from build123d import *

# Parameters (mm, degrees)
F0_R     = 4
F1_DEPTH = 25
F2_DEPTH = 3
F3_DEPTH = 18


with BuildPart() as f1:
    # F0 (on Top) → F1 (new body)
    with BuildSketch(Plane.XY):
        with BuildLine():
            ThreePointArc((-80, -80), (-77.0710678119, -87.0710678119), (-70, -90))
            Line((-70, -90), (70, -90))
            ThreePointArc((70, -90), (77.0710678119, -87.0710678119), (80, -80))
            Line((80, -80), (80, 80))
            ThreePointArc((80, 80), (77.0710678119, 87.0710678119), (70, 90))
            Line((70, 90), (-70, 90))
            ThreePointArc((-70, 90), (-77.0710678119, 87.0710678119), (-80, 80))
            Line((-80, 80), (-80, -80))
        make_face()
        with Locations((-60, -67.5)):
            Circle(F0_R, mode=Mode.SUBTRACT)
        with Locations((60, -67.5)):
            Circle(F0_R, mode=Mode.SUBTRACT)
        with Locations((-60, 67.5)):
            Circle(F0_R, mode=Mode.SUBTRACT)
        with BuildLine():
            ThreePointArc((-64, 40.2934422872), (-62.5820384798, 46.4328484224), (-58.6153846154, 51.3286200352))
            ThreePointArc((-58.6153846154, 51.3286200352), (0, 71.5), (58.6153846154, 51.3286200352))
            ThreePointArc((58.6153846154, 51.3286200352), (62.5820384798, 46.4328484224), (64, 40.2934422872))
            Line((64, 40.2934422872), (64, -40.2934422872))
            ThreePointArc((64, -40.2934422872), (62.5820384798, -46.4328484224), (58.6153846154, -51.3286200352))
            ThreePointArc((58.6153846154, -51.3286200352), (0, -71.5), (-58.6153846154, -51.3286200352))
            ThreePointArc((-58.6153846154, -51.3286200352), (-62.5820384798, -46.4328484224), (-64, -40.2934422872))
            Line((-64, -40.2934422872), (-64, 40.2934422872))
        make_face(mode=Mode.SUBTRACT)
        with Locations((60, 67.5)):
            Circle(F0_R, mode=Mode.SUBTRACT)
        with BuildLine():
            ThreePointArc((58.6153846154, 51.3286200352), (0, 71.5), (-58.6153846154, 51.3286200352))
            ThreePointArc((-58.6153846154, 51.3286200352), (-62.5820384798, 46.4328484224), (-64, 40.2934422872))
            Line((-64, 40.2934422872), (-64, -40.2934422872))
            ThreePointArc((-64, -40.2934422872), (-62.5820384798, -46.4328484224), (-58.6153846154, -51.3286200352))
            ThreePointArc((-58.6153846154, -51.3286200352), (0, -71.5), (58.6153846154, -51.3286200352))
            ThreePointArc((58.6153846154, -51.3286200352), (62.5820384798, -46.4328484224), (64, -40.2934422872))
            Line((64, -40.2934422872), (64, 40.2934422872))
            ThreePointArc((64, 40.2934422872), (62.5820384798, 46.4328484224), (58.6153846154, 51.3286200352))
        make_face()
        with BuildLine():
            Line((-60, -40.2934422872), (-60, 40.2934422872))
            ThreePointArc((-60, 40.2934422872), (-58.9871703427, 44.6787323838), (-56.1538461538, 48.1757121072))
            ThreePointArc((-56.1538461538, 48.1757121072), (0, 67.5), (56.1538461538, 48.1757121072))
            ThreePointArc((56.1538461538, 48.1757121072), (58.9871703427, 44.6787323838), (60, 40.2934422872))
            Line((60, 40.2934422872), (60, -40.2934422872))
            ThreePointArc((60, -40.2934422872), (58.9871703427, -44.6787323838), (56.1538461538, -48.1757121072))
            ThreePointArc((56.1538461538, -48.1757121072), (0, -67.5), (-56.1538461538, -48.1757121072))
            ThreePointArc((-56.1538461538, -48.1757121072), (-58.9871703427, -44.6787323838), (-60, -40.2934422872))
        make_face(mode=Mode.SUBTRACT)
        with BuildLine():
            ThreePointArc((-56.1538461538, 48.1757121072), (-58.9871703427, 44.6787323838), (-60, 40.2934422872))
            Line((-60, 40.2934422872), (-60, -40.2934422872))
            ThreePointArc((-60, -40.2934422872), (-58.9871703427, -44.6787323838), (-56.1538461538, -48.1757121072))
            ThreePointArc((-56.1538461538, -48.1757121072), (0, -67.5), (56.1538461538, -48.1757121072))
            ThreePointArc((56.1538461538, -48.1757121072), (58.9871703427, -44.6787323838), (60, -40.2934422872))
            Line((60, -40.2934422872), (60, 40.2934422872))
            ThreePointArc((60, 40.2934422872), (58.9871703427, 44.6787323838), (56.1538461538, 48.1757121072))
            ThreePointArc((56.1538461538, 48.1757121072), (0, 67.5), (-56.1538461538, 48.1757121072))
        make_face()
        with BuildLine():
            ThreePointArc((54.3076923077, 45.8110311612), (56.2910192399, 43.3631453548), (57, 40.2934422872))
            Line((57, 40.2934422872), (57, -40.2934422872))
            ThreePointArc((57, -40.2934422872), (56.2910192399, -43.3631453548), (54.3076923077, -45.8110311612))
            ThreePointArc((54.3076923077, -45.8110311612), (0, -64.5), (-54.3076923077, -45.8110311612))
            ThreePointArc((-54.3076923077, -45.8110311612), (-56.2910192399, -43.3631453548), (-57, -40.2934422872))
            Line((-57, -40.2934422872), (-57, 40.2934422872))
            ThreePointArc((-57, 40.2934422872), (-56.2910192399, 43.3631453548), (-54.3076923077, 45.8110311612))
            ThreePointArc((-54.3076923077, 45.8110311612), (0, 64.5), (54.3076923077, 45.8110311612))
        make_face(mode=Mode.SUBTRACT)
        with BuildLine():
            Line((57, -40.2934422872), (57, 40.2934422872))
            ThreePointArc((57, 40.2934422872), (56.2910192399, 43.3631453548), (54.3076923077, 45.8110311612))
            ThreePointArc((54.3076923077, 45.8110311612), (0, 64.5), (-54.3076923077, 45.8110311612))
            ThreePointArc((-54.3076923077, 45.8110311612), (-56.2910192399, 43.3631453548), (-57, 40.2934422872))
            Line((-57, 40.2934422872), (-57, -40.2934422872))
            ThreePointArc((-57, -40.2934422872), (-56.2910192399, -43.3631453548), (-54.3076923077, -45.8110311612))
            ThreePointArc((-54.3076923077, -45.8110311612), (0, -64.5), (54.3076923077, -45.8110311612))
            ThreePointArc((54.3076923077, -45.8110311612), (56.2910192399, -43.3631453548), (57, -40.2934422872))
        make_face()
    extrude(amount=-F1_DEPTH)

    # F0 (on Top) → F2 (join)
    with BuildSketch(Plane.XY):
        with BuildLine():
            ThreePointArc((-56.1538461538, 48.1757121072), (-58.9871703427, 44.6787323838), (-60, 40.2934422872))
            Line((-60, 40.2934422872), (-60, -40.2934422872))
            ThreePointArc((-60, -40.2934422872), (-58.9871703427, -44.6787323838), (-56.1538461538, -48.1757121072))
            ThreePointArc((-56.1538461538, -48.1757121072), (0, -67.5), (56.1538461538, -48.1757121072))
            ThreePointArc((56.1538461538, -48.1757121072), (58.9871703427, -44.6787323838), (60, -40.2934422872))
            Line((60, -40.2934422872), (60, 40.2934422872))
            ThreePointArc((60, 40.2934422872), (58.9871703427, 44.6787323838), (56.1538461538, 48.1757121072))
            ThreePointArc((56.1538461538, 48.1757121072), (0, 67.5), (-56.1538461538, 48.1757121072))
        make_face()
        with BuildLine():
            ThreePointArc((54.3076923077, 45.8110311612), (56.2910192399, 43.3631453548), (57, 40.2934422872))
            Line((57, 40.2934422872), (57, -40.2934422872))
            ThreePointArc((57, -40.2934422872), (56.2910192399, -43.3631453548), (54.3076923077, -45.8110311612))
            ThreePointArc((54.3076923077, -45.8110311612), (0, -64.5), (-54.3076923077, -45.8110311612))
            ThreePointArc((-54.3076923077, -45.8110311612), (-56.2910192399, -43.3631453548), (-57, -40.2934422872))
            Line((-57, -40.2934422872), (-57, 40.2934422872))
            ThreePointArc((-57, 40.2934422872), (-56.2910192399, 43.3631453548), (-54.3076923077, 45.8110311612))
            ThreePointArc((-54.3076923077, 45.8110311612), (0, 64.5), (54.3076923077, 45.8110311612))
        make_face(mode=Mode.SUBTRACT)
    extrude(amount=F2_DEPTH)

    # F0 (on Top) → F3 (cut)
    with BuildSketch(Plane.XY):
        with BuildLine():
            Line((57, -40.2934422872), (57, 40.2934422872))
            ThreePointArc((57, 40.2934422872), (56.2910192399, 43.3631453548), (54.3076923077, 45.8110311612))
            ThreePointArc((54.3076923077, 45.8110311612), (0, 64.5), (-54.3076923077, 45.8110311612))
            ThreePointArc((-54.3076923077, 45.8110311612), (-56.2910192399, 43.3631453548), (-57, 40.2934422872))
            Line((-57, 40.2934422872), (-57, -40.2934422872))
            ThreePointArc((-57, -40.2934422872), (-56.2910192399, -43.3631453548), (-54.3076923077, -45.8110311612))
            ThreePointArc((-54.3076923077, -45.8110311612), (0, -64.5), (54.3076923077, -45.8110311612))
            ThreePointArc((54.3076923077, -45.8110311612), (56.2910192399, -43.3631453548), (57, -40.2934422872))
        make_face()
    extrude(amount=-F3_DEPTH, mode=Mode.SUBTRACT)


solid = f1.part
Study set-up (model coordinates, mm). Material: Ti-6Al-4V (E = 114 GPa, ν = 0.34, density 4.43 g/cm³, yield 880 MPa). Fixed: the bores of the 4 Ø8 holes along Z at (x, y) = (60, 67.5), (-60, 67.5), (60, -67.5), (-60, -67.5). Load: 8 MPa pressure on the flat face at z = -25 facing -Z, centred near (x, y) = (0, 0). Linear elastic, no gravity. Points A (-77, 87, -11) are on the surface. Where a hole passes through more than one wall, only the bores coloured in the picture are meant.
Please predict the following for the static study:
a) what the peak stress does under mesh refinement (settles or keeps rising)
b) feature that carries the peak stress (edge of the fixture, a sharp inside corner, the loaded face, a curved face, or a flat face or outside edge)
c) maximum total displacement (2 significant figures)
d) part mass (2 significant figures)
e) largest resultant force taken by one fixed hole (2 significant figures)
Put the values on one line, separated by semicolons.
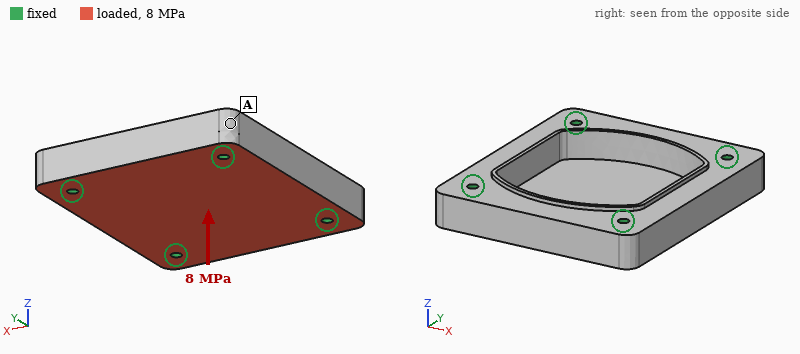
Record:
keeps rising; edge of the fixture; 0.92 mm; 2.1 kg; 60 kN
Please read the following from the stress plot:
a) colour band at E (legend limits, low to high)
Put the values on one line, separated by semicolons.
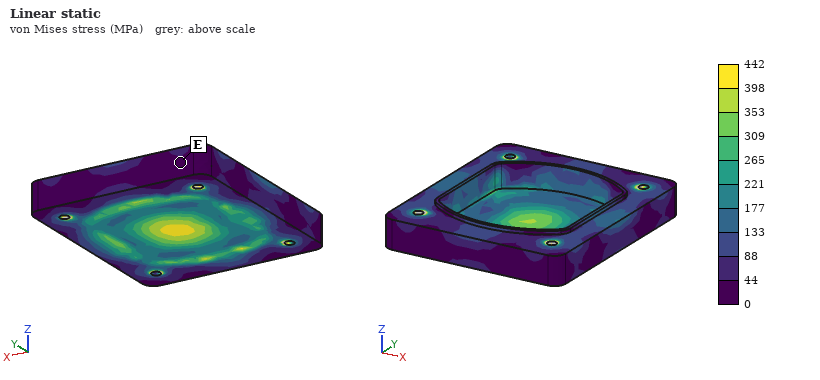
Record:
0 to 44 MPa
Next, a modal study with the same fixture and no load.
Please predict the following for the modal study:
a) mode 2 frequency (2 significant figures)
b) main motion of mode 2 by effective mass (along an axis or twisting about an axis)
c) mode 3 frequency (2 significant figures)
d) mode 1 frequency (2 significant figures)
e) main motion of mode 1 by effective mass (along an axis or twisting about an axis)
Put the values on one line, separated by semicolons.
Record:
5500 Hz; twisting about Y; 6000 Hz; 3400 Hz; along Z
